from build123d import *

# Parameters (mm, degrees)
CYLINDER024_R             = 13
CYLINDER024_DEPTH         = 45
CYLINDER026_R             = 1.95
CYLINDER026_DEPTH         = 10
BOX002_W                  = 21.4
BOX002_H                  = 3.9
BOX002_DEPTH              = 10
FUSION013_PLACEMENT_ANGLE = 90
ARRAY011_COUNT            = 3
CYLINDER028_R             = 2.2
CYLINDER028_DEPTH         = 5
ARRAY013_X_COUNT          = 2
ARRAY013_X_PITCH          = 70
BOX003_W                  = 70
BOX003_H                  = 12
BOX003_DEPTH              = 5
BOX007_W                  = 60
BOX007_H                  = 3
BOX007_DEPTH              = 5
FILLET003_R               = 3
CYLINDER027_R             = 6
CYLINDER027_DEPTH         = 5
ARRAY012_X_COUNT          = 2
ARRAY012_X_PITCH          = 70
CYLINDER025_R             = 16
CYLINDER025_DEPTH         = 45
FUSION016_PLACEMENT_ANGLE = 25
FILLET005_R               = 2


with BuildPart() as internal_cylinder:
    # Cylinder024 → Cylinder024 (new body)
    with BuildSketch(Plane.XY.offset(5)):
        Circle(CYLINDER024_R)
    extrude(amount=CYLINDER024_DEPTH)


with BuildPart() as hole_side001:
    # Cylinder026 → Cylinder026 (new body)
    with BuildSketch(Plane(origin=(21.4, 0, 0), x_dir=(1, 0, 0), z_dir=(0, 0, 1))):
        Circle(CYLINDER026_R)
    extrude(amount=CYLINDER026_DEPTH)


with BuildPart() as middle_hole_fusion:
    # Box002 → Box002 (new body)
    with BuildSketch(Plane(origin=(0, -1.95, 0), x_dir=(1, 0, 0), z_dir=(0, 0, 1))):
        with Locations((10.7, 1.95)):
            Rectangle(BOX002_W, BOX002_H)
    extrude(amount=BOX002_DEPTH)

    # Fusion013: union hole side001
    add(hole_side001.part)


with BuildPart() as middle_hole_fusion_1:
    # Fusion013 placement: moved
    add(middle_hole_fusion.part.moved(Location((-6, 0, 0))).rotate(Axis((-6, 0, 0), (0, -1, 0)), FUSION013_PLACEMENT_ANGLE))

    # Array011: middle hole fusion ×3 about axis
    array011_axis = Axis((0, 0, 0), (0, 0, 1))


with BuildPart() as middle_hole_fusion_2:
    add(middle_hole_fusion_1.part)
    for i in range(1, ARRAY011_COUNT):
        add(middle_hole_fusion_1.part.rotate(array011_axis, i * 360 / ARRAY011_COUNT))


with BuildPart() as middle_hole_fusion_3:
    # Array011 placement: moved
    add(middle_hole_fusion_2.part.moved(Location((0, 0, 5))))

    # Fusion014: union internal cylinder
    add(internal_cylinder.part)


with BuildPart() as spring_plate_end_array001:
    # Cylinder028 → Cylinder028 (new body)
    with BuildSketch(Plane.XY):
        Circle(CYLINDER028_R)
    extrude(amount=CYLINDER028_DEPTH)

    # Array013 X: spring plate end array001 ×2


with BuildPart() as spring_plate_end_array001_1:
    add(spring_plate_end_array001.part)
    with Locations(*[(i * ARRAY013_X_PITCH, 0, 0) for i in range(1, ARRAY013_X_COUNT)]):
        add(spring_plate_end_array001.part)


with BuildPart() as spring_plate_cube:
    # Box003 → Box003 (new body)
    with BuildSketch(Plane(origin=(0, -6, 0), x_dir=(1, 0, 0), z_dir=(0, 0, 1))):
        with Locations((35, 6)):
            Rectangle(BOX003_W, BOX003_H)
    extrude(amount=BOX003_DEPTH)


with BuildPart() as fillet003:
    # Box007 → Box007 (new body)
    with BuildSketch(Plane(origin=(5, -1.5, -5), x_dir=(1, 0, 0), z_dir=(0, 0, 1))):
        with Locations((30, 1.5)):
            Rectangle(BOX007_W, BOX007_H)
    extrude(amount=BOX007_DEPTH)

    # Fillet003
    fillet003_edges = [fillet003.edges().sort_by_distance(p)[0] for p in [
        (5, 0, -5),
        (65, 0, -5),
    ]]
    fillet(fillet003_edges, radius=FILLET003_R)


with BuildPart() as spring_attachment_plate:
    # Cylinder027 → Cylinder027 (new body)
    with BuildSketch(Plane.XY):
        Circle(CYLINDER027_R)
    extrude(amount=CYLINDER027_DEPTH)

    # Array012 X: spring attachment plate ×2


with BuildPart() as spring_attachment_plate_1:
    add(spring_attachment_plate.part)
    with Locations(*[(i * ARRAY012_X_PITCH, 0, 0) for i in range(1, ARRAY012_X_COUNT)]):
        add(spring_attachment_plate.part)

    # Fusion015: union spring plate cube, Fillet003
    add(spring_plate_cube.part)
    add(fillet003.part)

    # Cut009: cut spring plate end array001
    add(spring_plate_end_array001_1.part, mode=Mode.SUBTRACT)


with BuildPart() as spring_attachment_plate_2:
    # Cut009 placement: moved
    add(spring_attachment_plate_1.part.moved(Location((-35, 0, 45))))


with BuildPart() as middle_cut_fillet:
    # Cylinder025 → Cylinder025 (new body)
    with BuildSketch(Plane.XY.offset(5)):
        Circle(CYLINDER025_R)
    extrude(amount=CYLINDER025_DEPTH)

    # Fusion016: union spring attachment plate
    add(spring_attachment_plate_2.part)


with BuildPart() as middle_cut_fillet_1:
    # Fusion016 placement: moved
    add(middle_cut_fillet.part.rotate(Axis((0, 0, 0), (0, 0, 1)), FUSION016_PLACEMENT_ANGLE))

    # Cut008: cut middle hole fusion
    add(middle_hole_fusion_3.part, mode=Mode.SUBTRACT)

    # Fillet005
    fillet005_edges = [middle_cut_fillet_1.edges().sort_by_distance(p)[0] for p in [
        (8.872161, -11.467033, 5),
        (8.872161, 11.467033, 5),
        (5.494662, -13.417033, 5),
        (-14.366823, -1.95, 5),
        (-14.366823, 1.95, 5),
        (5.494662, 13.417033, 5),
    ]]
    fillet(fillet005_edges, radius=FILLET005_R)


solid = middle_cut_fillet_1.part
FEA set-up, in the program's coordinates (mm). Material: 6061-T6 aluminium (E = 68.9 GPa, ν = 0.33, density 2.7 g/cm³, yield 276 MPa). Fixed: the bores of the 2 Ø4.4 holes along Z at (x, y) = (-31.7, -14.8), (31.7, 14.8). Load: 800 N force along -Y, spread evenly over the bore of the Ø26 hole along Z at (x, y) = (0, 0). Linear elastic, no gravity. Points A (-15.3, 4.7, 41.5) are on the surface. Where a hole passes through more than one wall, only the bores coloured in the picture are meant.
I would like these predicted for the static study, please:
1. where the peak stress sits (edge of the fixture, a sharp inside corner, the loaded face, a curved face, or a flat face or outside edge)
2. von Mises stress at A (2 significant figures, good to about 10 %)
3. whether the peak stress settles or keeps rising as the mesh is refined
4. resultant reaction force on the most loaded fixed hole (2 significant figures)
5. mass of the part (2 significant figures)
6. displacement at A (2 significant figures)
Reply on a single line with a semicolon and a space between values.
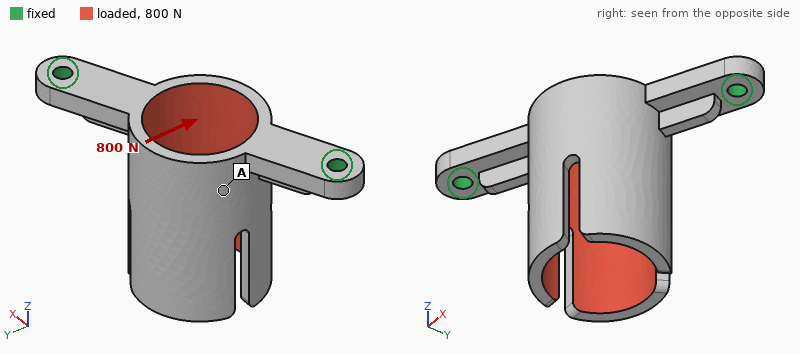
edge of the fixture; 17 MPa; keeps rising; 420 N; 39 g; 0.15 mm
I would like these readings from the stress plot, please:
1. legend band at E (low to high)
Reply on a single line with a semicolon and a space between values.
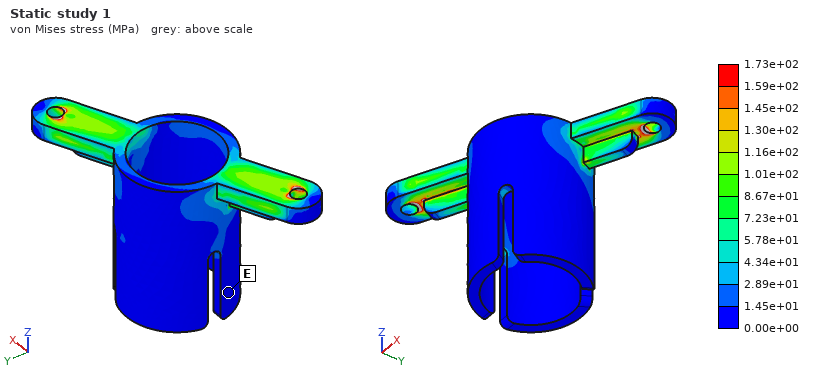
0.00e+00 to 1.45e+01 MPa
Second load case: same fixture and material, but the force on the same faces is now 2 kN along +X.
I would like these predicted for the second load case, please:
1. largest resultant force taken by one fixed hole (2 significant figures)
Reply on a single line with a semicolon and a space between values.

1.2 kN
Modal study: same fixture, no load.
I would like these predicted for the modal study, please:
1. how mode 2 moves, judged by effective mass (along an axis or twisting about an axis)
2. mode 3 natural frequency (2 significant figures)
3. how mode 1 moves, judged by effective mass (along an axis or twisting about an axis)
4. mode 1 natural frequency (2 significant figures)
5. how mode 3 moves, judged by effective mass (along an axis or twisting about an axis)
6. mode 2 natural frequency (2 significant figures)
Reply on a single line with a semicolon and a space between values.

along Z; 3800 Hz; along Y; 1200 Hz; along X; 3300 Hz
